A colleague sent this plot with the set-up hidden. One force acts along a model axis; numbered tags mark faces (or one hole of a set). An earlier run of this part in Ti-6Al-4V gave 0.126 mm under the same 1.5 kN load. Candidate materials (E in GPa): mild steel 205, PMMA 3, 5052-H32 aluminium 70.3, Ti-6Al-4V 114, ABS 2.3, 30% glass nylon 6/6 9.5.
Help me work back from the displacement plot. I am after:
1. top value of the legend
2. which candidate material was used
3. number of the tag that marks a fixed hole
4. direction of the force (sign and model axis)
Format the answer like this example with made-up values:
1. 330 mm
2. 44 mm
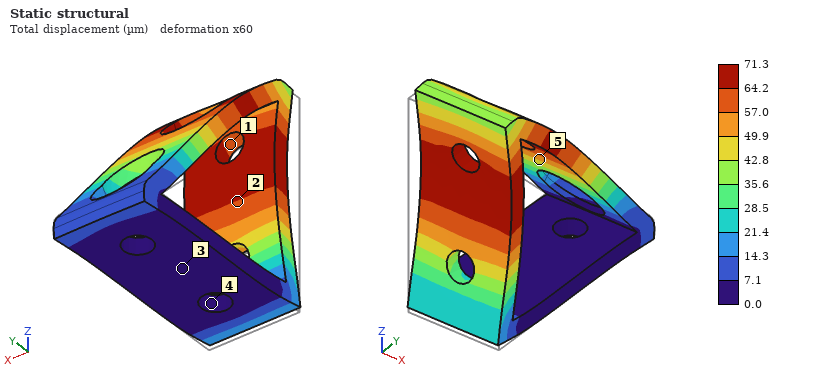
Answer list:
1. 71.3 µm
2. mild steel
3. 4
4. +Y
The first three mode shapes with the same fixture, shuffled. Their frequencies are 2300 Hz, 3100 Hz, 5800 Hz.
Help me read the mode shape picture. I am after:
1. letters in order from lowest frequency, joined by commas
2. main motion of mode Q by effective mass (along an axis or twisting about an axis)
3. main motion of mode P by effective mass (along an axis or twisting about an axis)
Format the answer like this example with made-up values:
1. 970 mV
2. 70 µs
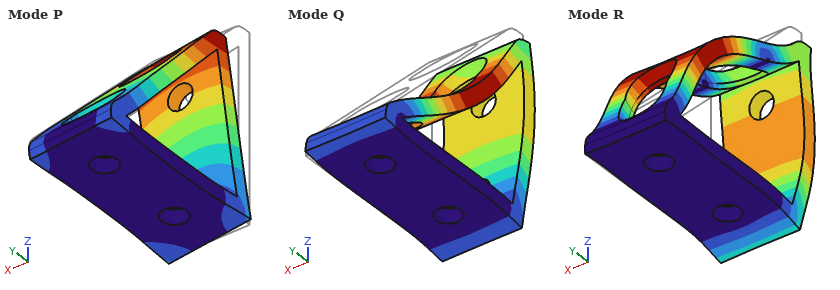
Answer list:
1. P, Q, R
2. along Y
3. along X
